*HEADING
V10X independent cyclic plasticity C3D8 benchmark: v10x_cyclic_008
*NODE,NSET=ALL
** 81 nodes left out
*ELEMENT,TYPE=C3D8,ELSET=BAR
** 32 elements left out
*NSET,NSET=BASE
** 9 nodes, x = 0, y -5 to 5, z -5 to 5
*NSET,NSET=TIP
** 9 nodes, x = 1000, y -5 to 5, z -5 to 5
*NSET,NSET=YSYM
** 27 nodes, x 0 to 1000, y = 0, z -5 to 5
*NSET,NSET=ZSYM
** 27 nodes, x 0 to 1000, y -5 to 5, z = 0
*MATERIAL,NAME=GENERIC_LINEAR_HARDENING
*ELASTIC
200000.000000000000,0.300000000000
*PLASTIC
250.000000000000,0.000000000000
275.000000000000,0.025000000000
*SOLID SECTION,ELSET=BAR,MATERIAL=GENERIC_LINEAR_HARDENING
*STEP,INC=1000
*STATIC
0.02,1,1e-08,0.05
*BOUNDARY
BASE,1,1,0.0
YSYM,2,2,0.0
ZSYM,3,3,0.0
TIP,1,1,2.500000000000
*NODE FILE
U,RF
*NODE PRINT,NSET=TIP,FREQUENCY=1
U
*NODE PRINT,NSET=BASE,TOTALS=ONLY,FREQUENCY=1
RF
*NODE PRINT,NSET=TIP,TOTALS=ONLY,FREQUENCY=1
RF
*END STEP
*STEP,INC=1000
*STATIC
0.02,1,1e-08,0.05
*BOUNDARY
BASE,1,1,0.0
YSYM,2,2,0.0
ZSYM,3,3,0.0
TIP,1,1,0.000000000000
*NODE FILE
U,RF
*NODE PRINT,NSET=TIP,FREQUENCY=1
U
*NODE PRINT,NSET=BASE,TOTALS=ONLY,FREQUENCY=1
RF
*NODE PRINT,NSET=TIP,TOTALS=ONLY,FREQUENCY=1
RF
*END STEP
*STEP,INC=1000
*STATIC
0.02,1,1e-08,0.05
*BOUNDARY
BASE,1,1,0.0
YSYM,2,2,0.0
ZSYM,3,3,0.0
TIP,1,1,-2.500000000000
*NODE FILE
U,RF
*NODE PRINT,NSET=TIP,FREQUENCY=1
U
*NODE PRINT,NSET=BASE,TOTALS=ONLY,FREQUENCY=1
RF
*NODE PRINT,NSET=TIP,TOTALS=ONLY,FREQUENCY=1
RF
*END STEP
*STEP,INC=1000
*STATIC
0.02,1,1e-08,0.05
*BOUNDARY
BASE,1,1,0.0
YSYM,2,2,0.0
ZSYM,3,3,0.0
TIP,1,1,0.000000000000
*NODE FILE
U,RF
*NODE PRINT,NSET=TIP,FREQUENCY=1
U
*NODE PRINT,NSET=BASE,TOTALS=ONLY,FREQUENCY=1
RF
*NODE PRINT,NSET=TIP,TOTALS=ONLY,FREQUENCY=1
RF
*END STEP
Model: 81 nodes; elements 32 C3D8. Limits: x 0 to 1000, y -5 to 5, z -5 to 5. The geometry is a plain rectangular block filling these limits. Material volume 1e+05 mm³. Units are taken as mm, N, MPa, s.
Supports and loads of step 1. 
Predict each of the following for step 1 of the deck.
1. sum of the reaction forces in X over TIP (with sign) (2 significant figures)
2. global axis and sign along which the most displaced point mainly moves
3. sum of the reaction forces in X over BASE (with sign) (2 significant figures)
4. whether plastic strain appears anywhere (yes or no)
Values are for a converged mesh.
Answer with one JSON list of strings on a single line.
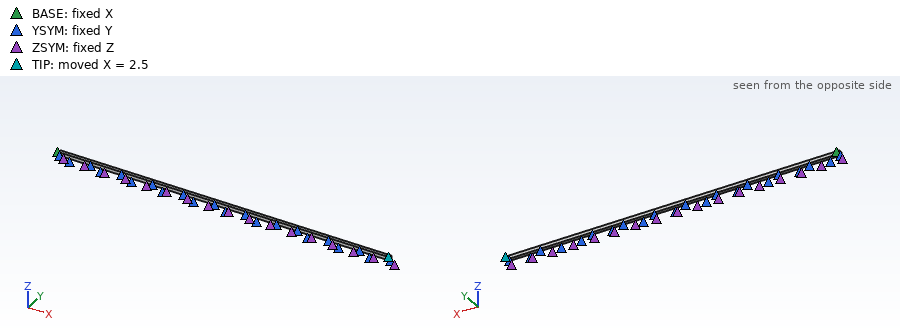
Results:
["25000 N", "+X", "-25000 N", "yes"]
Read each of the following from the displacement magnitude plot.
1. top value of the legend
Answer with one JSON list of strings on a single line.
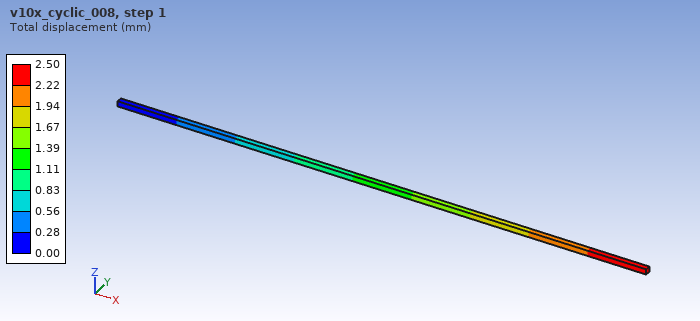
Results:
["2.50 mm"]
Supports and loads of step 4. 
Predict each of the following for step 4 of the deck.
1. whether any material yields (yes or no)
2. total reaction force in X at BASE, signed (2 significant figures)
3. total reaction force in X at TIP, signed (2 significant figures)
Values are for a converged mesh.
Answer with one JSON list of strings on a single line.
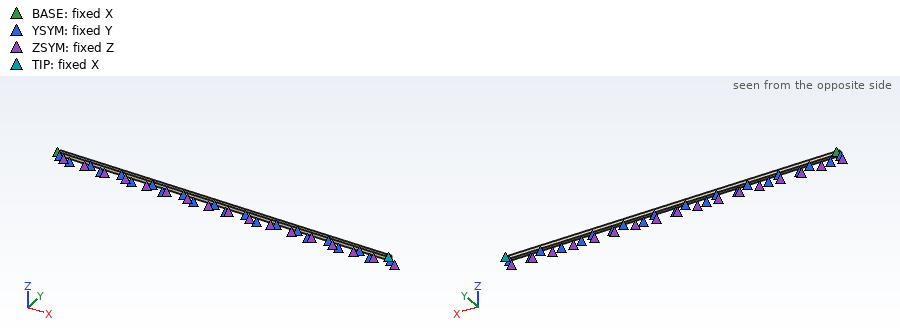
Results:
["yes", "-25000 N", "25000 N"]
